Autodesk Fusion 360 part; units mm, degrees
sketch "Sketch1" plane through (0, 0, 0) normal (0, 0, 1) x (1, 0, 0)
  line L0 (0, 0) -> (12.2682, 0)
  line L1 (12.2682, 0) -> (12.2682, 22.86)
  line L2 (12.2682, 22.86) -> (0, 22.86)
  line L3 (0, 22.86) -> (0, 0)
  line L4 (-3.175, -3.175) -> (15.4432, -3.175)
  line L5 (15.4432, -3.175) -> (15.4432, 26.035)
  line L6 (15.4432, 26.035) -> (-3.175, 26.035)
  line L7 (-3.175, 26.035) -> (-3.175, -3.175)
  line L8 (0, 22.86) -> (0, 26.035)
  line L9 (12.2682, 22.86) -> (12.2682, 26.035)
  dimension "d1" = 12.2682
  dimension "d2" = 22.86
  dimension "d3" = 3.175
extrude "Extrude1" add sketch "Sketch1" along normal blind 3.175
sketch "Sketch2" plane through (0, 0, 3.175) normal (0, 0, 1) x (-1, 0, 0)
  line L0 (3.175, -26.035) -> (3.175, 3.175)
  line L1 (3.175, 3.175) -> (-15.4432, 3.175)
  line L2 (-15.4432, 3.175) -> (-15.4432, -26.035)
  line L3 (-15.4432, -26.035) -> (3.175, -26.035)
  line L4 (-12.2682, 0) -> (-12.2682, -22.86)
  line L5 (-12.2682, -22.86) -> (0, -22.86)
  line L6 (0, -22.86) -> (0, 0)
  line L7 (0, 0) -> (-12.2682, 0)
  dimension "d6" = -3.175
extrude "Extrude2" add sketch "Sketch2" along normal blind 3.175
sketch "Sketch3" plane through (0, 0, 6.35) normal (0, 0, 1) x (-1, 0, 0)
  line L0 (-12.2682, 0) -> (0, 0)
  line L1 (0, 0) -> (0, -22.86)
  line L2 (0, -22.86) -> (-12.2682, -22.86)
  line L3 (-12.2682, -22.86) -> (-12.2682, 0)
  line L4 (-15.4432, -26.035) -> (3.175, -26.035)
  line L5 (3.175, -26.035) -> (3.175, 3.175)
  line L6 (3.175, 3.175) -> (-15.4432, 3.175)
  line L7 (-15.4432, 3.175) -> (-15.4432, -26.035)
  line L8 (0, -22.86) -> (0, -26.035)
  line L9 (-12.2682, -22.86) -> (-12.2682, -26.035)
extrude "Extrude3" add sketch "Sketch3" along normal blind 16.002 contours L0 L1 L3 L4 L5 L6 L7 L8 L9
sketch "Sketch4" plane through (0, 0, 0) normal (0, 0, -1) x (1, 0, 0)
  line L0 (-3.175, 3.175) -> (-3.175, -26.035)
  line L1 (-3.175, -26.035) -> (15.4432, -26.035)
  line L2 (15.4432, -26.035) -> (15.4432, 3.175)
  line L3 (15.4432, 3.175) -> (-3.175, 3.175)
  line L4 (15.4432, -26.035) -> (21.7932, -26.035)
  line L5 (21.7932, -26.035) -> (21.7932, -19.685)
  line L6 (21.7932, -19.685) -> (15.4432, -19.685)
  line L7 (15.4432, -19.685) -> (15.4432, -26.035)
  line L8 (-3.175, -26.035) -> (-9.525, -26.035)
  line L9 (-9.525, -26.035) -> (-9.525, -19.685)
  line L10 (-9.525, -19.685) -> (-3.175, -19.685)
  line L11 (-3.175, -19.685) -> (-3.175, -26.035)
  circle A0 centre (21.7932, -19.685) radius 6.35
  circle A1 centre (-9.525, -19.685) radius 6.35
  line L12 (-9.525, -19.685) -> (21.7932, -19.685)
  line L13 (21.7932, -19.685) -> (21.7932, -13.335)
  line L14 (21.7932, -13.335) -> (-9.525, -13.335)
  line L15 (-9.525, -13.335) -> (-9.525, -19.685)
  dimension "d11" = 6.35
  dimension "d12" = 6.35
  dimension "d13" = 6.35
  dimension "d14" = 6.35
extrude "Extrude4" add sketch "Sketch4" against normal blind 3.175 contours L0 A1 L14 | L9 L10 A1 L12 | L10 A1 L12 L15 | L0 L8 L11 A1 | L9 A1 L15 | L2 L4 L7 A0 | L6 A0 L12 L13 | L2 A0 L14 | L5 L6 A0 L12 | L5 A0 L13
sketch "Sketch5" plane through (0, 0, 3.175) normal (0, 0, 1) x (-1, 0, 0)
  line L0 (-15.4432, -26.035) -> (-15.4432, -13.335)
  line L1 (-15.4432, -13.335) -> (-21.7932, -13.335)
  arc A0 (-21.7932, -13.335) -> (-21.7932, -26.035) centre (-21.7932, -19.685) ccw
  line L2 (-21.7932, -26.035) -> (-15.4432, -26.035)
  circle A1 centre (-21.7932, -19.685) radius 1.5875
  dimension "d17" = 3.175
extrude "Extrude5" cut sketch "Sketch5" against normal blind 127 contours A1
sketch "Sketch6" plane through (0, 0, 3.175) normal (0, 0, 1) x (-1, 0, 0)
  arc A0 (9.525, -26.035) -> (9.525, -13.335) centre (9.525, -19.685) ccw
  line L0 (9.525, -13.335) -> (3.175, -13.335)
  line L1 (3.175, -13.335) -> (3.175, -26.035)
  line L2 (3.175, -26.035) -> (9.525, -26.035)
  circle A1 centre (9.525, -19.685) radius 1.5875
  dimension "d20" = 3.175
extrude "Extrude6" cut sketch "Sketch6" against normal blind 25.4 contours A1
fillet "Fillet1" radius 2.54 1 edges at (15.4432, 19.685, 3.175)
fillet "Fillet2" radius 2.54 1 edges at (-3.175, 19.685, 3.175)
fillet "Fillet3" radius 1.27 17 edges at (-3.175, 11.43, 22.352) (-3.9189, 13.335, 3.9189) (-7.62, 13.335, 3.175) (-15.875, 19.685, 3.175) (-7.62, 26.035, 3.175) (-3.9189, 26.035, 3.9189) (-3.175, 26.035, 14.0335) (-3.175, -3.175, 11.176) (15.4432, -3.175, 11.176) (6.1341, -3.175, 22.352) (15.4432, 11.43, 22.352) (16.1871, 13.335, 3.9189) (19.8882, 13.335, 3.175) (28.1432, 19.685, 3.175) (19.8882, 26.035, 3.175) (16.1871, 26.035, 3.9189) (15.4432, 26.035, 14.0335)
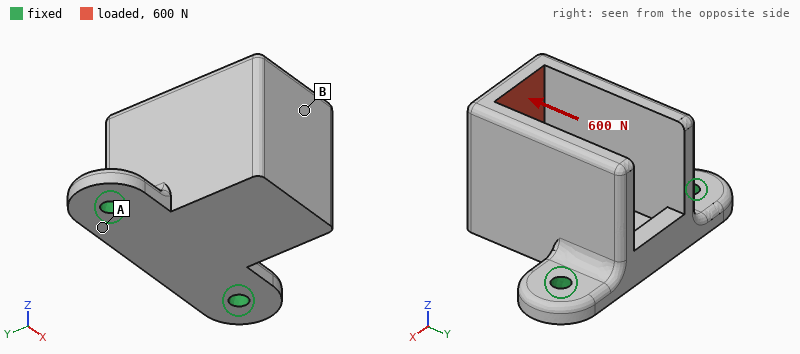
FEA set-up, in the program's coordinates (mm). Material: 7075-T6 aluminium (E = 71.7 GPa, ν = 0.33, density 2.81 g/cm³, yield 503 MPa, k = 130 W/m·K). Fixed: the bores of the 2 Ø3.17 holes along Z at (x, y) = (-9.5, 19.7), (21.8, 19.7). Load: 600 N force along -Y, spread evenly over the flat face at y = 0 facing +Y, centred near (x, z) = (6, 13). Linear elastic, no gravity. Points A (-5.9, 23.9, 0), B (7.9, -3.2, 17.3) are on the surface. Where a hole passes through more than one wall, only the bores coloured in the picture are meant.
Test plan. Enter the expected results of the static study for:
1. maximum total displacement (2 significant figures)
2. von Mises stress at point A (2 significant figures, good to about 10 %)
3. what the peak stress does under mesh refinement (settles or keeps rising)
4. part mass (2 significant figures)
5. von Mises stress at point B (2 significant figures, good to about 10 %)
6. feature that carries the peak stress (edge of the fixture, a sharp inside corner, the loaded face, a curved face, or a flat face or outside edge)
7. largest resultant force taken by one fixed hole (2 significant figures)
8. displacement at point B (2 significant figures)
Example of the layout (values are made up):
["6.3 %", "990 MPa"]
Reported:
["0.17 mm", "56 MPa", "keeps rising", "20 g", "22 MPa", "edge of the fixture", "300 N", "0.15 mm"]
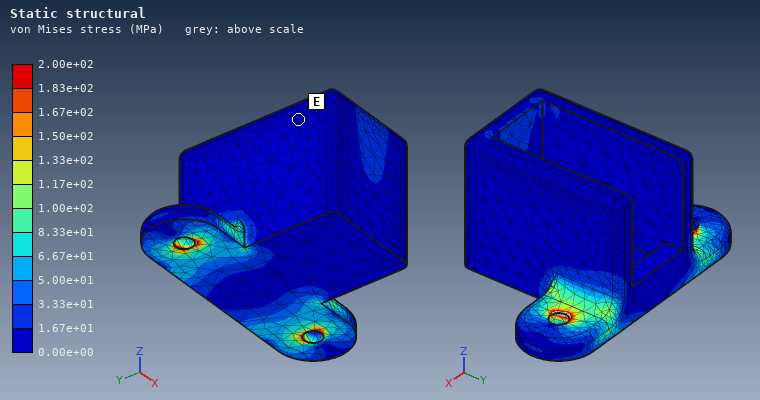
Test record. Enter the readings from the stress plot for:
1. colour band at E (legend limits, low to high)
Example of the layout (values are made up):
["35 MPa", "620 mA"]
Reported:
["0.00e+00 to 1.67e+01 MPa"]
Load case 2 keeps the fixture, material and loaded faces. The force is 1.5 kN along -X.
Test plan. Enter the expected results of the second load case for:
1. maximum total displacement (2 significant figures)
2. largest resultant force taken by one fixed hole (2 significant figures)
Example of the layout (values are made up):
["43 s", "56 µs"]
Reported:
["0.20 mm", "1.4 kN"]
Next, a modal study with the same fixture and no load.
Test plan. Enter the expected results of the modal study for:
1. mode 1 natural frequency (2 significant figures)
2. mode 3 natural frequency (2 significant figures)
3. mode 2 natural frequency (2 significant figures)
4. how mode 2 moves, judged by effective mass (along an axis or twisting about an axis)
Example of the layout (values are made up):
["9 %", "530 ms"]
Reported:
["2600 Hz", "8400 Hz", "5500 Hz", "along X"]
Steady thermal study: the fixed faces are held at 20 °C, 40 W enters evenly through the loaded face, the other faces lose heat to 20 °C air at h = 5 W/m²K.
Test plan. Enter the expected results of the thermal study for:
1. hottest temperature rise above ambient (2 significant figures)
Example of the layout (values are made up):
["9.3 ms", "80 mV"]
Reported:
["81 K"]
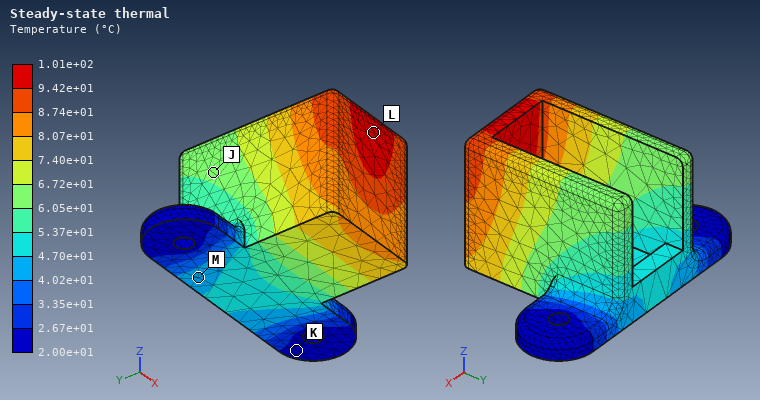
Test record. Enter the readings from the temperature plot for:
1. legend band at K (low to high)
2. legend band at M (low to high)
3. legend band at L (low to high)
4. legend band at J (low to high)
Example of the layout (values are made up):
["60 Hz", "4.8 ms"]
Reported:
["2.00e+01 to 2.67e+01 °C", "4.02e+01 to 4.70e+01 °C", "9.42e+01 to 1.01e+02 °C", "6.05e+01 to 6.72e+01 °C"]
